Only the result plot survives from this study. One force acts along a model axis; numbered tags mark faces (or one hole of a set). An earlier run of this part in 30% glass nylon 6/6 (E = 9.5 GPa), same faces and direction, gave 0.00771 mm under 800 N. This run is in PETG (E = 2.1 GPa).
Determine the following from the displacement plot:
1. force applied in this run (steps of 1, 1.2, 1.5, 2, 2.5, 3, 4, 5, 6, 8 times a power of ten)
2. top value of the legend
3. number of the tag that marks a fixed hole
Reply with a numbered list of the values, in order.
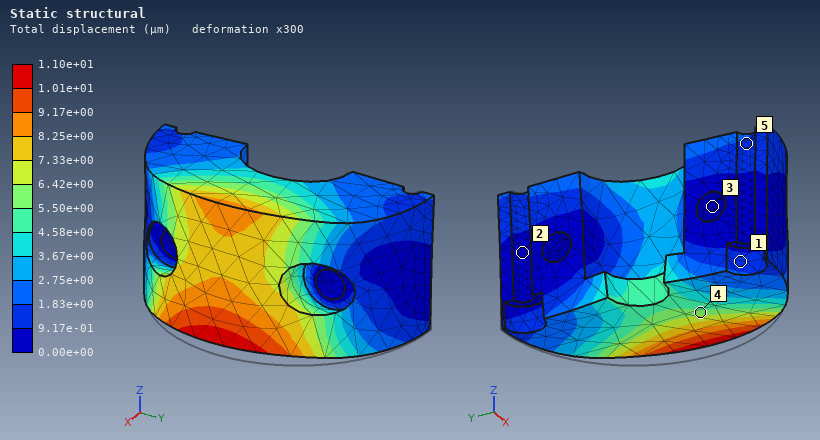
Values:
1. 250 N
2. 1.10e+01 µm
3. 3
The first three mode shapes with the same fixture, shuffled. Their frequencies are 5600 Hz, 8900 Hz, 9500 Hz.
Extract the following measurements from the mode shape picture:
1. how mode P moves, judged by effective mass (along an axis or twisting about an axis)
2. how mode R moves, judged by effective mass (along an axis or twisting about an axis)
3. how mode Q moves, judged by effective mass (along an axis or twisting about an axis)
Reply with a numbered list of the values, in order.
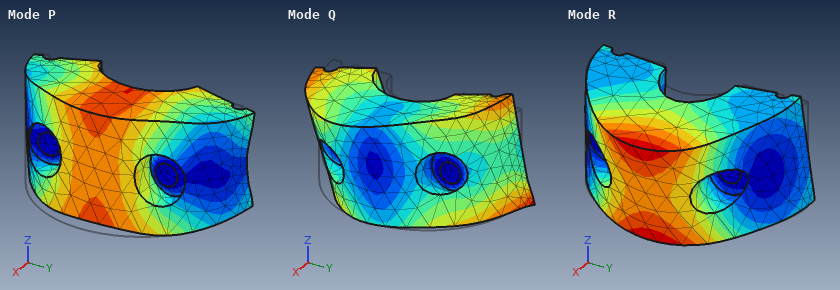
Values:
1. along X
2. along Z
3. twisting about X
